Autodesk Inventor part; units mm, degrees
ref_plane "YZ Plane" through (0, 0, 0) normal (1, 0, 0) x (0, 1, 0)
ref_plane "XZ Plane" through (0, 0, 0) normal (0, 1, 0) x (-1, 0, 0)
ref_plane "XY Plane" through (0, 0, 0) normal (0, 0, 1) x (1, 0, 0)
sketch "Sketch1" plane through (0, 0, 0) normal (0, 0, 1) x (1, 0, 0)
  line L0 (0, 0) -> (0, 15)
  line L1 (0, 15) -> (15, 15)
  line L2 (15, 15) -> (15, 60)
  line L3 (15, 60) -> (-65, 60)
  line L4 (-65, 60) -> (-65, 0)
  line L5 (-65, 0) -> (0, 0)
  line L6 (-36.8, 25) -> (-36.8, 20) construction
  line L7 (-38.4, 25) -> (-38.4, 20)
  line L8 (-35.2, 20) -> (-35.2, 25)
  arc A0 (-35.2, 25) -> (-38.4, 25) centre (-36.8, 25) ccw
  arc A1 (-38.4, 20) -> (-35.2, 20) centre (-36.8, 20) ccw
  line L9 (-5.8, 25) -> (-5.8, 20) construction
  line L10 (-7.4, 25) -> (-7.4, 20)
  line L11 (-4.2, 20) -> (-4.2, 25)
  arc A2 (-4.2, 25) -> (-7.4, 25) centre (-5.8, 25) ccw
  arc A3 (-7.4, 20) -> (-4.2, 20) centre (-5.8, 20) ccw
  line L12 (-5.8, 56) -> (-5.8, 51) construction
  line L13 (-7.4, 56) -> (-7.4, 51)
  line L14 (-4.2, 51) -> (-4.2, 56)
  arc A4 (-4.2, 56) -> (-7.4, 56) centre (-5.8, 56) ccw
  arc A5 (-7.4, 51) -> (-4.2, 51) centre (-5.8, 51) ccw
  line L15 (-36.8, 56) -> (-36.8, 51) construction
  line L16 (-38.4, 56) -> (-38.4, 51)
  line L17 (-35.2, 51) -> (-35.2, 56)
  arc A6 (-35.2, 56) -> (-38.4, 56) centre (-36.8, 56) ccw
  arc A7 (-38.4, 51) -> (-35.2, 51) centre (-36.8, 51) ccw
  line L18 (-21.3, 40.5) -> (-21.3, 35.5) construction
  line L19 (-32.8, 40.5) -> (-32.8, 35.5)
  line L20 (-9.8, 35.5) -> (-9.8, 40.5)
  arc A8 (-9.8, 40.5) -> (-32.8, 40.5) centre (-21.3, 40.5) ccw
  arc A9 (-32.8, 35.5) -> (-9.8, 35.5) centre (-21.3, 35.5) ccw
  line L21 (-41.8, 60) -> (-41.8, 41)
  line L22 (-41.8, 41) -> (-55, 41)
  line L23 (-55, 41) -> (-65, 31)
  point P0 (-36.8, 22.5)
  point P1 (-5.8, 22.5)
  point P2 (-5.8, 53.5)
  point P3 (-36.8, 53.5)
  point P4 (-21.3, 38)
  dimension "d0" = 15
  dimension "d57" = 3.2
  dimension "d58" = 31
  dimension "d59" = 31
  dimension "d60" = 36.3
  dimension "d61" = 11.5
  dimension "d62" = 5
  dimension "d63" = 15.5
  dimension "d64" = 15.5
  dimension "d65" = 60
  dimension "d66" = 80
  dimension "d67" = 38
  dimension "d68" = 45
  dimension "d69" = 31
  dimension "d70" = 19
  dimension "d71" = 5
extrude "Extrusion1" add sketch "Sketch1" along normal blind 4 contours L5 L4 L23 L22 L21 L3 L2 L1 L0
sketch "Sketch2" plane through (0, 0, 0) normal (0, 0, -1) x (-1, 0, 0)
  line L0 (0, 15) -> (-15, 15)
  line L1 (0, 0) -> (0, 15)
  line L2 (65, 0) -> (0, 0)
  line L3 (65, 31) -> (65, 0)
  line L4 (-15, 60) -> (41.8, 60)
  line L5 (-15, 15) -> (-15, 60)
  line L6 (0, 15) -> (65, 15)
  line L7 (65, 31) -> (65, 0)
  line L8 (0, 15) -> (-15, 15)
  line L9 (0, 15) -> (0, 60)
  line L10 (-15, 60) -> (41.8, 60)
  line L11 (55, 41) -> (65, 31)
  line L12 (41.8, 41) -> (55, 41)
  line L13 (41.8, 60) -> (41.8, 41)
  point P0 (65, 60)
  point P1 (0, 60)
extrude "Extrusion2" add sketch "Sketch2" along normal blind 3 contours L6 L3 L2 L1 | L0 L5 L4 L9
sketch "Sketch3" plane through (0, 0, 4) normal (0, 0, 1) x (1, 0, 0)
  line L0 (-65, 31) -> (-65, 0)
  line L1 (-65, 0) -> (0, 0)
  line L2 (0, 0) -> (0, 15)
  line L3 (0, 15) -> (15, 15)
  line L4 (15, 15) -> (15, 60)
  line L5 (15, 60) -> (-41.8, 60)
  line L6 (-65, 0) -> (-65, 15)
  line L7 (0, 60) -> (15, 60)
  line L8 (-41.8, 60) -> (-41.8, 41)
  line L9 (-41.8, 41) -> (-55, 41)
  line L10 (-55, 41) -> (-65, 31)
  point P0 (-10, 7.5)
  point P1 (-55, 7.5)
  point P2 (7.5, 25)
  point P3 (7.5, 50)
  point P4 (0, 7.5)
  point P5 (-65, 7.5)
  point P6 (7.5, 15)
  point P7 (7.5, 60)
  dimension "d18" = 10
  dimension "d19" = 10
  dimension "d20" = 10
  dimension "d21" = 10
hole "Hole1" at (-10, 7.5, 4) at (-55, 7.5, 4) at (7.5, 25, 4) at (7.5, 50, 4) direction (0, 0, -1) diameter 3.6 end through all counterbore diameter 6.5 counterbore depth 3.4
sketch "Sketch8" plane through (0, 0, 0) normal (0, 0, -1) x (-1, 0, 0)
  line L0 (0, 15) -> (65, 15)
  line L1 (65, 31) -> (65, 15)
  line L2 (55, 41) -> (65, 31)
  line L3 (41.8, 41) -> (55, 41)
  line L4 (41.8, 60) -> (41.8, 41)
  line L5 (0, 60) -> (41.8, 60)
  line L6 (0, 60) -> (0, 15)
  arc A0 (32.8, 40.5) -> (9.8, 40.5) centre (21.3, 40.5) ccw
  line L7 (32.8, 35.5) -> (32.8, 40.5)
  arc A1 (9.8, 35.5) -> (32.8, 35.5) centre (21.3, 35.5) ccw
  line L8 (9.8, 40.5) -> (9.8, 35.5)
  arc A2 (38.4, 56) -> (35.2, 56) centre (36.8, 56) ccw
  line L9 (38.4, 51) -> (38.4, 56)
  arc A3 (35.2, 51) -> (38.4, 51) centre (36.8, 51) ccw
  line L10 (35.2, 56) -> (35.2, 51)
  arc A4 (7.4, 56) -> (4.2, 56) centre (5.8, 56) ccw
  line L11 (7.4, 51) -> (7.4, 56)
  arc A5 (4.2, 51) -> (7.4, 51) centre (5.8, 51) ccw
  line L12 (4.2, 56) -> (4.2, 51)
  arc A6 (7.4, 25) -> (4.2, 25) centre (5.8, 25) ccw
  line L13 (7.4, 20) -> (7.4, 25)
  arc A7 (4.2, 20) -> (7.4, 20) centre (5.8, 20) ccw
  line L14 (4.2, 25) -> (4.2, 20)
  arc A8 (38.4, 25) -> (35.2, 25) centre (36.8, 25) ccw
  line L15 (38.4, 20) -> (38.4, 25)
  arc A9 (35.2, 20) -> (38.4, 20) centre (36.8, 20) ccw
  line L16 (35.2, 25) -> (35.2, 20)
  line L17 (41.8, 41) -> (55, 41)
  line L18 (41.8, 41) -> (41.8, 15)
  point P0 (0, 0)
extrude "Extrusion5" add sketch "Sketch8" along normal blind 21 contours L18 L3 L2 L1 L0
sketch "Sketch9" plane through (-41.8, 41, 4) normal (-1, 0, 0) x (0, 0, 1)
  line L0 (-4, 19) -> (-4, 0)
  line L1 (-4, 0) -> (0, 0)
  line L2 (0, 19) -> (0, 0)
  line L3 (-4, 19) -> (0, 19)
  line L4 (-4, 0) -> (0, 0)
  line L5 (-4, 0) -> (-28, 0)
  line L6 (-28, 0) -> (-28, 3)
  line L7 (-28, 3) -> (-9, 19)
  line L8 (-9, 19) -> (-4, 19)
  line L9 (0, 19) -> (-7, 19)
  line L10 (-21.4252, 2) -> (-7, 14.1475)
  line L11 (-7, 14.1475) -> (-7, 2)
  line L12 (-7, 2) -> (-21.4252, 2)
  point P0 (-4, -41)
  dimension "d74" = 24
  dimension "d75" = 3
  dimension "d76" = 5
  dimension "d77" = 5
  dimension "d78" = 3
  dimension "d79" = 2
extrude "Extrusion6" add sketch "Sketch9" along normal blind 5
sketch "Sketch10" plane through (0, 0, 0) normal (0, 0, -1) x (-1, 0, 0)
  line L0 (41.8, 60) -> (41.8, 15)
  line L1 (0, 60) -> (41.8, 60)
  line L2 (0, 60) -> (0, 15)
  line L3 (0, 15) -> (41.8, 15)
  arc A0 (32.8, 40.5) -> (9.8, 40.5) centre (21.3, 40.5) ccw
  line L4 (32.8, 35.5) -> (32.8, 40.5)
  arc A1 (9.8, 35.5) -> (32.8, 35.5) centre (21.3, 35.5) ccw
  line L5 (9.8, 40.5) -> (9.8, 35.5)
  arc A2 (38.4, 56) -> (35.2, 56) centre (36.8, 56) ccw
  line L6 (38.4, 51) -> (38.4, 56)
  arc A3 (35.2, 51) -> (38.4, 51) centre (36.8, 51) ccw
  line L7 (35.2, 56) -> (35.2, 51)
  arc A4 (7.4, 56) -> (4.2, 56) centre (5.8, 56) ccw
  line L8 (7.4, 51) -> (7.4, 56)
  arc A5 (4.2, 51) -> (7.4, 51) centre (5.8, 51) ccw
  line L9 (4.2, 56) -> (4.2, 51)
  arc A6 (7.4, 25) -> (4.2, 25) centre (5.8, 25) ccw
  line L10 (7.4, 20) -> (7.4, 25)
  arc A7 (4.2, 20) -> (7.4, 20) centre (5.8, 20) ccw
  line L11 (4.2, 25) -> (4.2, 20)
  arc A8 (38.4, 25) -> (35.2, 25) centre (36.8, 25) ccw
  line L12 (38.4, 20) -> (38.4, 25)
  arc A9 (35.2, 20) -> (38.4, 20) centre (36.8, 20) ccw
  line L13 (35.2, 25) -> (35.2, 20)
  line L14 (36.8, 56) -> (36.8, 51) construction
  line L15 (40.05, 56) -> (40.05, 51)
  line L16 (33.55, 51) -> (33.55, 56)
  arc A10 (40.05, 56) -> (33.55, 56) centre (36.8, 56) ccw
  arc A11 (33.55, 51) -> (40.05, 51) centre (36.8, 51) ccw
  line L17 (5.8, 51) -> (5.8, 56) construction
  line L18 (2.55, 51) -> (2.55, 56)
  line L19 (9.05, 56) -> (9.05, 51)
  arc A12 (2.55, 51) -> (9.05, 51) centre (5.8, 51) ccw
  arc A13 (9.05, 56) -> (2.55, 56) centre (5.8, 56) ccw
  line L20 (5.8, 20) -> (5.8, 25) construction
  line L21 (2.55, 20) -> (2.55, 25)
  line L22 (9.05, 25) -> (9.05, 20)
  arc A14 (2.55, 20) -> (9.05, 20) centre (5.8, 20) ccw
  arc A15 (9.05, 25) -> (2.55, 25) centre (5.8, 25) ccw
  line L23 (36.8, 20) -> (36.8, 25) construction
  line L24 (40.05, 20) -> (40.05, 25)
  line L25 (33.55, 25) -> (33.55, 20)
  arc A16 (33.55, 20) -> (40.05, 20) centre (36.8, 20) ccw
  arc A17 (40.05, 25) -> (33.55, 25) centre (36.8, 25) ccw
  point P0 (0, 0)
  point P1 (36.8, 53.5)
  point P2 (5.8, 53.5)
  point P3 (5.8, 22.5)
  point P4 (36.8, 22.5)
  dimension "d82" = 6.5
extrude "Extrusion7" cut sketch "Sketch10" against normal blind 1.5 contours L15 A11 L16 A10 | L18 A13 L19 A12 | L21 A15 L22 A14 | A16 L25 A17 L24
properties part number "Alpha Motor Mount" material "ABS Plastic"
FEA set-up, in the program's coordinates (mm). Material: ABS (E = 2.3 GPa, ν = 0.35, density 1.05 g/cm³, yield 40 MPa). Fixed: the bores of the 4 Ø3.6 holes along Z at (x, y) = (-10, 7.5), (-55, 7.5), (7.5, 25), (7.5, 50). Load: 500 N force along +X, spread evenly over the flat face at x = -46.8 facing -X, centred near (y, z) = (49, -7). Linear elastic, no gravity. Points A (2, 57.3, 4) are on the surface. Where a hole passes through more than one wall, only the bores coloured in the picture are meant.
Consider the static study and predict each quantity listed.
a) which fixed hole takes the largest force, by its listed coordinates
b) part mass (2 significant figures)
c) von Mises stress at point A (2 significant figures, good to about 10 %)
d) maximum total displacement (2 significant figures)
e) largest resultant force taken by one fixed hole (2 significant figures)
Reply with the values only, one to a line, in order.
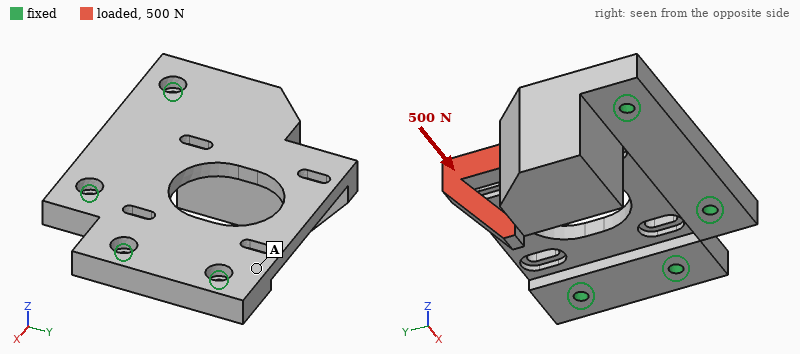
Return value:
(-55, 7.5)
33 g
6.0 MPa
1.0 mm
370 N
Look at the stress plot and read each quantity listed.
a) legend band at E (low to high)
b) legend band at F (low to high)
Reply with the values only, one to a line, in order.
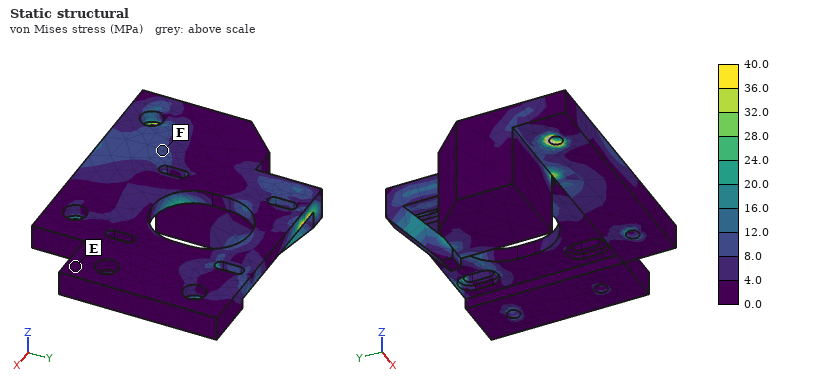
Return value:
0.0 to 4.0 MPa
8.0 to 12.0 MPa
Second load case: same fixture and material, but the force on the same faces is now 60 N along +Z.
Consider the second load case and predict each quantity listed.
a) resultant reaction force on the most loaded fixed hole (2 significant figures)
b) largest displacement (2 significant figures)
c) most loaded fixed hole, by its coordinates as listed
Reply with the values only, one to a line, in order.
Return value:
68 N
1.1 mm
(-55, 7.5)
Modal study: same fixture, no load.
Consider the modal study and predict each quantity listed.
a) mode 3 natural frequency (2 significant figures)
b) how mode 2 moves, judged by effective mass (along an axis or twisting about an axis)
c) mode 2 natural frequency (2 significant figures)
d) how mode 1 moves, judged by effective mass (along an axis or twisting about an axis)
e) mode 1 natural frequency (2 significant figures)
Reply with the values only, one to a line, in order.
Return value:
2400 Hz
along X
1200 Hz
along Z
500 Hz
